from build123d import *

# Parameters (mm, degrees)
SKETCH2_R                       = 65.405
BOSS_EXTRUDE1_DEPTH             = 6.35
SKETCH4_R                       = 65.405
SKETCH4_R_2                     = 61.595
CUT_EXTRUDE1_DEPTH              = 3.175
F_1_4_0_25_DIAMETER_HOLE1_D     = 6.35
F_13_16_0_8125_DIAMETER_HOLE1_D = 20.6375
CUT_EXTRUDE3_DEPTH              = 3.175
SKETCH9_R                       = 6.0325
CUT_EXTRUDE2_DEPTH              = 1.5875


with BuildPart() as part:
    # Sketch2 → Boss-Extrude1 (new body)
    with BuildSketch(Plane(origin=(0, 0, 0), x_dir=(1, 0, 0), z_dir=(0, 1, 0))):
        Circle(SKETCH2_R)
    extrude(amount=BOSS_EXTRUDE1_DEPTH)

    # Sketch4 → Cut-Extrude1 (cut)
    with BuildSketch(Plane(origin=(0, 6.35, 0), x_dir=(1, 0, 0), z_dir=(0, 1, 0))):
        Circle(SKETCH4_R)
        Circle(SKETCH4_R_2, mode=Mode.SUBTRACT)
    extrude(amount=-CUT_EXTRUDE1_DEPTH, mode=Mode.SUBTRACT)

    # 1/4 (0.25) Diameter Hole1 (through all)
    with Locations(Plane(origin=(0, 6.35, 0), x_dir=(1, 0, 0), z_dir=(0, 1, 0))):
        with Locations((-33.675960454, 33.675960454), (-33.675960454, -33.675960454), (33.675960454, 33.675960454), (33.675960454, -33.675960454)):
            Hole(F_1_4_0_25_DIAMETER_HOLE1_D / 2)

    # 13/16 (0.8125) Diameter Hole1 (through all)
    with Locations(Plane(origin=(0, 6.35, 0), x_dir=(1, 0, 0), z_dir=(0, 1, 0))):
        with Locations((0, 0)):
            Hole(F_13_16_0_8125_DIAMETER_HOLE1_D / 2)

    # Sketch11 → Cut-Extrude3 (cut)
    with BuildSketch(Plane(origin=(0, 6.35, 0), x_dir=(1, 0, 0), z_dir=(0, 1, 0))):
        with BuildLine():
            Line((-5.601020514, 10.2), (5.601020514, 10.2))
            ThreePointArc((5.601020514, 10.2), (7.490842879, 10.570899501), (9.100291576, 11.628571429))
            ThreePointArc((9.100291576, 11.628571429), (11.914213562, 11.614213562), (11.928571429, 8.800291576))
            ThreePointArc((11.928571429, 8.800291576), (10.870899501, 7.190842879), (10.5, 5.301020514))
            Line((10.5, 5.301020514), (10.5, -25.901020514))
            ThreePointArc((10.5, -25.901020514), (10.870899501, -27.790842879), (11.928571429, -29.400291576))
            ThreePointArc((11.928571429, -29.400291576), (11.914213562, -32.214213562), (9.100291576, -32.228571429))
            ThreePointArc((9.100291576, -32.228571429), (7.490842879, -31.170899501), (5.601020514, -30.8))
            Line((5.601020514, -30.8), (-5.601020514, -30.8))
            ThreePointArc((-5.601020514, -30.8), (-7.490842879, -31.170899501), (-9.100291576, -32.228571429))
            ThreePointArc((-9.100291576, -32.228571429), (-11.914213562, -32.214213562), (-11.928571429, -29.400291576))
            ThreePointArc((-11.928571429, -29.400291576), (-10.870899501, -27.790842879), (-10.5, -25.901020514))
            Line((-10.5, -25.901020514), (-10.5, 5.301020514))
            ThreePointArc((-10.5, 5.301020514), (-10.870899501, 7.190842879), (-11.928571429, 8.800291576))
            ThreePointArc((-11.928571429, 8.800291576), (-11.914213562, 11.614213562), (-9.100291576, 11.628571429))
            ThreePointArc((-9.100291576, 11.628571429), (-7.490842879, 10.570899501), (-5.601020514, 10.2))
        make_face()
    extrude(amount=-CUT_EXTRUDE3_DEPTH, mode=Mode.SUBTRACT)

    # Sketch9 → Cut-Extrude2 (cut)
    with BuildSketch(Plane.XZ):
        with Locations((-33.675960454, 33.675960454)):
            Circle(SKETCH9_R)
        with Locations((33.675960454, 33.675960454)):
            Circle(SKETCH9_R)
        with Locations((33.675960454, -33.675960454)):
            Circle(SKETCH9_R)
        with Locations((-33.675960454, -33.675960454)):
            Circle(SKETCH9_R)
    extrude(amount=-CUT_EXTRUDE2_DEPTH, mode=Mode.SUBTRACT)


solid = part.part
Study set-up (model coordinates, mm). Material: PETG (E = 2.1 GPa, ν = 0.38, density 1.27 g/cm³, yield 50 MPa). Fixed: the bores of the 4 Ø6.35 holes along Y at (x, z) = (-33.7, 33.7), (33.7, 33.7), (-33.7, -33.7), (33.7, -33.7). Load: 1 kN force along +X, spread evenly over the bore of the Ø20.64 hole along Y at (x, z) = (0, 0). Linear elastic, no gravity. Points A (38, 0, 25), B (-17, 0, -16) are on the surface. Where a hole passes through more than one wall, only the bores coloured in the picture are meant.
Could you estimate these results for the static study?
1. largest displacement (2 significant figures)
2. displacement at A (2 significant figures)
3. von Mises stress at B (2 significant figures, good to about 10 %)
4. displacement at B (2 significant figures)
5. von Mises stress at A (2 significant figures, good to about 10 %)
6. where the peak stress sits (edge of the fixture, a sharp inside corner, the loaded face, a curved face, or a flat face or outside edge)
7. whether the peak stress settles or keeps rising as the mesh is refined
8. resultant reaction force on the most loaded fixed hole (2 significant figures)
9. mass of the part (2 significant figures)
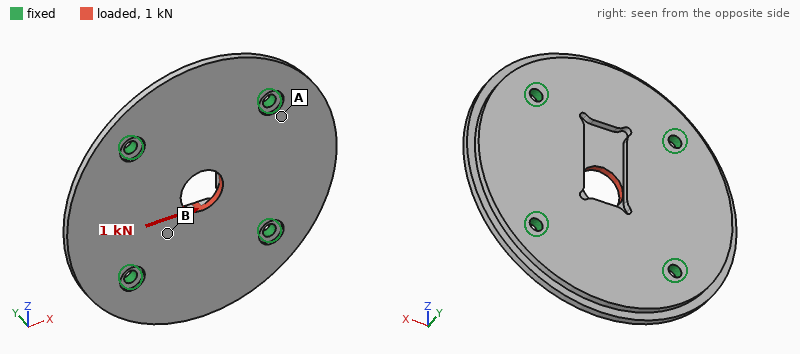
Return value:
76 µm
16 µm
2.4 MPa
30 µm
1.2 MPa
a sharp inside corner
keeps rising
280 N
96 g
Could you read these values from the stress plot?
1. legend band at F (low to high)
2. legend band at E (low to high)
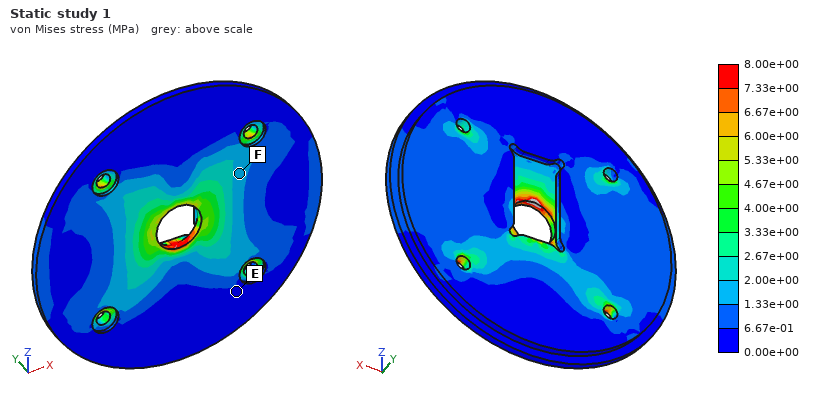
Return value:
1.33e+00 to 2.00e+00 MPa
0.00e+00 to 6.67e-01 MPa
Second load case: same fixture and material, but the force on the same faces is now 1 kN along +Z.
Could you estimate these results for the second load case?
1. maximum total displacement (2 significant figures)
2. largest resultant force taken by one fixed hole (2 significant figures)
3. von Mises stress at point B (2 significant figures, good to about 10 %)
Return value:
63 µm
270 N
2.2 MPa
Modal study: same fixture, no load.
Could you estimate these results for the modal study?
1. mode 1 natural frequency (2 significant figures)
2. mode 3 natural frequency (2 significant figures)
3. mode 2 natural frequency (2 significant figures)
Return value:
960 Hz
1100 Hz
1100 Hz
